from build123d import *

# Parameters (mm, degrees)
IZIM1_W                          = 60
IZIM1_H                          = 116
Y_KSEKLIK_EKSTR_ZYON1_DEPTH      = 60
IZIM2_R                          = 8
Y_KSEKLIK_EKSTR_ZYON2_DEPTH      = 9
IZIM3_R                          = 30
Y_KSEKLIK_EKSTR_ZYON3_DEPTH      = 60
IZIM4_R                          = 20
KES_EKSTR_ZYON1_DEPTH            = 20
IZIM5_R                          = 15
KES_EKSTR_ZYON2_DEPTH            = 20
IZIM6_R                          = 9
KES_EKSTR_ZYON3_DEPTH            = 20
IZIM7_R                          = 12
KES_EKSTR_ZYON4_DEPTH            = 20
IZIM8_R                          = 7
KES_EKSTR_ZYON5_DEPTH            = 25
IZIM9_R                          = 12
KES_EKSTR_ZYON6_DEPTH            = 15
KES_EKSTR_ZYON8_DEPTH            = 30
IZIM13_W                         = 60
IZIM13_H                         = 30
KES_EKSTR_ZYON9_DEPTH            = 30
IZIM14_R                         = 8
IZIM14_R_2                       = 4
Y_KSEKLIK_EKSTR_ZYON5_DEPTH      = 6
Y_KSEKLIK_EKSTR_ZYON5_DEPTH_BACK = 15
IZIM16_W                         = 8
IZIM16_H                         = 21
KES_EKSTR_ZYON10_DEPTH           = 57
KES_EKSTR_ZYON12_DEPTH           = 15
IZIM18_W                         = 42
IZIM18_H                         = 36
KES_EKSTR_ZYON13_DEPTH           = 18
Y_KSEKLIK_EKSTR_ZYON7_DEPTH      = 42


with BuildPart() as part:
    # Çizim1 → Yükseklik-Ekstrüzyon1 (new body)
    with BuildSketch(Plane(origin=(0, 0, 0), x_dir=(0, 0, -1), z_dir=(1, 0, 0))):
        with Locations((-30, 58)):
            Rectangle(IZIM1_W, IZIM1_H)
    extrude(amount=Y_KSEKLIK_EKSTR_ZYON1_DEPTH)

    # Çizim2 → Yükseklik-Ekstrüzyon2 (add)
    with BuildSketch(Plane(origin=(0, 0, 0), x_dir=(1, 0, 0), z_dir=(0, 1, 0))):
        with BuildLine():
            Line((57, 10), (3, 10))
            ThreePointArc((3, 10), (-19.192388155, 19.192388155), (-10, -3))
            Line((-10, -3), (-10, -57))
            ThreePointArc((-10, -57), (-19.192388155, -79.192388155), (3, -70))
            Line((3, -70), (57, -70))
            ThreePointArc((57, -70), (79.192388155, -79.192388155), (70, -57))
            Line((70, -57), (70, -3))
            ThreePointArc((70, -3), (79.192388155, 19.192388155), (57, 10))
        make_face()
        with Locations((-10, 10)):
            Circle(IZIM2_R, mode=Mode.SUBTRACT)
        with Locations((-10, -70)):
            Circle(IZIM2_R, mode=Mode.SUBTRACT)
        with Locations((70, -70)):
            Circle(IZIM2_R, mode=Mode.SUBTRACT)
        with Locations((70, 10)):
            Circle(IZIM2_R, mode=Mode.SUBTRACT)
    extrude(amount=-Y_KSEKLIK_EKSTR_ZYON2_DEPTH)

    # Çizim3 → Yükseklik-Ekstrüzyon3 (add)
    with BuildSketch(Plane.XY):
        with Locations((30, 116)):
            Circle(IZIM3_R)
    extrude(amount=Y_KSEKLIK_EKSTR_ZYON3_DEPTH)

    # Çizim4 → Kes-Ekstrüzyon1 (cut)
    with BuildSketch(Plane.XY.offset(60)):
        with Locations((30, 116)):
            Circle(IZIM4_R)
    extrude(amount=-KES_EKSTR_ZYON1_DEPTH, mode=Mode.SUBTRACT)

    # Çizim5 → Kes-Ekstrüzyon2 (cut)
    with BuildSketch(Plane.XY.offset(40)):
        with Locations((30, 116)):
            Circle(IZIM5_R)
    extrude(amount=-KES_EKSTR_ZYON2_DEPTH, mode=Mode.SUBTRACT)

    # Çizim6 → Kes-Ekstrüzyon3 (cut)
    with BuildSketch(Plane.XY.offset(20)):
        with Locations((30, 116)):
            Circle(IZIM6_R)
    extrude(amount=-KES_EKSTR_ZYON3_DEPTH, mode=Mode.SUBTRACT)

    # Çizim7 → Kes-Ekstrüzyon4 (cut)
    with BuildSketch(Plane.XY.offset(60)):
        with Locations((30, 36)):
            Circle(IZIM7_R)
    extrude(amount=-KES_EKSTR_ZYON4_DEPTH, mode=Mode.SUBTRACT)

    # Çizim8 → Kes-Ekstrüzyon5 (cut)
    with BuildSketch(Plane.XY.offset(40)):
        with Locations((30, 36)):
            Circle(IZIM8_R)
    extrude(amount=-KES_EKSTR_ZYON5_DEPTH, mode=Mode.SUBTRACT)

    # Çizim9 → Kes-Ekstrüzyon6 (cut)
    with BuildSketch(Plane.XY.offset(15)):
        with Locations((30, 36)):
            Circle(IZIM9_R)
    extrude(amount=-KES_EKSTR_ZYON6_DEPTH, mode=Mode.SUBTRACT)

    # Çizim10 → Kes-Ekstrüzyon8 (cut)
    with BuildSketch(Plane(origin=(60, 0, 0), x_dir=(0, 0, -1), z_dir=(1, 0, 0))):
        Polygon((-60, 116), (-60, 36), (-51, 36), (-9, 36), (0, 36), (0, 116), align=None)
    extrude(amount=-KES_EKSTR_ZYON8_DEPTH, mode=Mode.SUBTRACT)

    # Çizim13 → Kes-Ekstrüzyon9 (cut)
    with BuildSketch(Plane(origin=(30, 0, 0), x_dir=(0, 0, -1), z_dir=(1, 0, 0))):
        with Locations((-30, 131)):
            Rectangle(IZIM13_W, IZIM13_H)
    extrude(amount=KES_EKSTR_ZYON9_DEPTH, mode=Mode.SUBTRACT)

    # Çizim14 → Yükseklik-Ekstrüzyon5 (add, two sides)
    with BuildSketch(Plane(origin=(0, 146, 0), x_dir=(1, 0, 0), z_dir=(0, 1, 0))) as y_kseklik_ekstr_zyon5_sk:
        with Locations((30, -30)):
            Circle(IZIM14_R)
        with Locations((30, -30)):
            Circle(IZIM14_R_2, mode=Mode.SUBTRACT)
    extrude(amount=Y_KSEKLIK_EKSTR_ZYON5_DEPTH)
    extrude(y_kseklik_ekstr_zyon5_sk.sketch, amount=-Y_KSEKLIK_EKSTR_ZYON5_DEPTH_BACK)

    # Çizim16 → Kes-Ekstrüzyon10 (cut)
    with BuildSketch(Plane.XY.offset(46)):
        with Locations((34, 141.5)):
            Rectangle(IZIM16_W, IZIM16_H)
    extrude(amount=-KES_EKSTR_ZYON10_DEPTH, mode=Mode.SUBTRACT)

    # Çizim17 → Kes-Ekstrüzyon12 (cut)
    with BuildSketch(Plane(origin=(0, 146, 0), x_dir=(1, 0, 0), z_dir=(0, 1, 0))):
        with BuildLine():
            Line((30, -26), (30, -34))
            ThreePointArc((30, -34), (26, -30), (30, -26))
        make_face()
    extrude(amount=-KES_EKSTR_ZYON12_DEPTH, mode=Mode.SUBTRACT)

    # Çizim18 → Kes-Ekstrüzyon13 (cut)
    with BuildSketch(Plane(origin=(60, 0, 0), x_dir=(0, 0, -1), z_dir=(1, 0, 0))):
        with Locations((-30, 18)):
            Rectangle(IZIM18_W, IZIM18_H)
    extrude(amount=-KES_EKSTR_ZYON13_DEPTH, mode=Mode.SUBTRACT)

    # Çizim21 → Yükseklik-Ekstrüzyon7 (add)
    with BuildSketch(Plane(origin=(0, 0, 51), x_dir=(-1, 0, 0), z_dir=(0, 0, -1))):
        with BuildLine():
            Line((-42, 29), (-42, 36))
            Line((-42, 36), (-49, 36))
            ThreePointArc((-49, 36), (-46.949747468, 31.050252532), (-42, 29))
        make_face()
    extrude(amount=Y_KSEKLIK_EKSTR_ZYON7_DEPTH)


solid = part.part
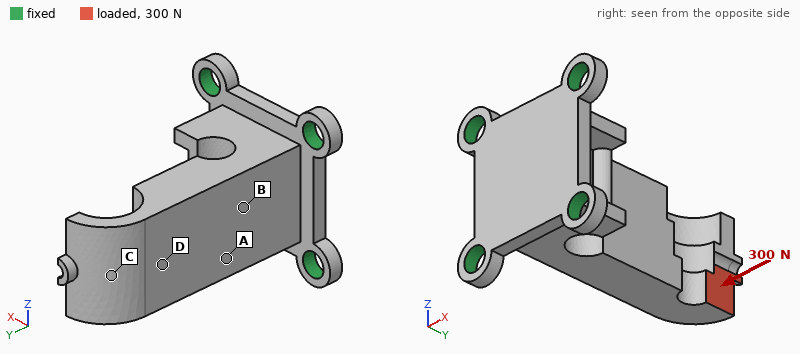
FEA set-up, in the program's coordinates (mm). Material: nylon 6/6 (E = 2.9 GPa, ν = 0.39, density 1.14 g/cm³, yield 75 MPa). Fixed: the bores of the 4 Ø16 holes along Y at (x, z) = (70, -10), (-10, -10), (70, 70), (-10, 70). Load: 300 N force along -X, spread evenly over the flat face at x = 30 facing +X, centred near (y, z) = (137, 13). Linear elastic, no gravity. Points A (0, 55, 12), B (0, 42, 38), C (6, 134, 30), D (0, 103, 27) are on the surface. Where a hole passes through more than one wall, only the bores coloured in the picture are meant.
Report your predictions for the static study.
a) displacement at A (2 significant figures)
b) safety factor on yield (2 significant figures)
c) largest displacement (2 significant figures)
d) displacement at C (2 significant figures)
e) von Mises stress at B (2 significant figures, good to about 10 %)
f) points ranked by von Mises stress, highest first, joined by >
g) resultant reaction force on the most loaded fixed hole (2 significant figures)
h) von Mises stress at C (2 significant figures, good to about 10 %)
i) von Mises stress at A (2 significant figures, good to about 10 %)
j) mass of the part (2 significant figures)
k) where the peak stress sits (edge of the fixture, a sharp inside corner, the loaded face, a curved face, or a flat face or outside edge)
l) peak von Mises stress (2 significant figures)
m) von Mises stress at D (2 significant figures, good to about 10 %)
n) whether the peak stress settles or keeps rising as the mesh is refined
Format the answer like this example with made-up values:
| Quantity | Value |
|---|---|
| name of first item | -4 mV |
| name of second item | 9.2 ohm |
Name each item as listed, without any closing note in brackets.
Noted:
| Quantity | Value |
|---|---|
| displacement at A | 0.33 mm |
| safety factor on yield | 5.3 |
| largest displacement | 1.5 mm |
| displacement at C | 1.2 mm |
| von Mises stress at B | 5.3 MPa |
| points ranked by von Mises stress, highest first, joined by > | B > A > D > C |
| resultant reaction force on the most loaded fixed hole | 380 N |
| von Mises stress at C | 0.96 MPa |
| von Mises stress at A | 3.4 MPa |
| mass of the part | 360 g |
| where the peak stress sits | a curved face |
| peak von Mises stress | 14 MPa |
| von Mises stress at D | 2.3 MPa |
| whether the peak stress settles or keeps rising as the mesh is refined | settles |
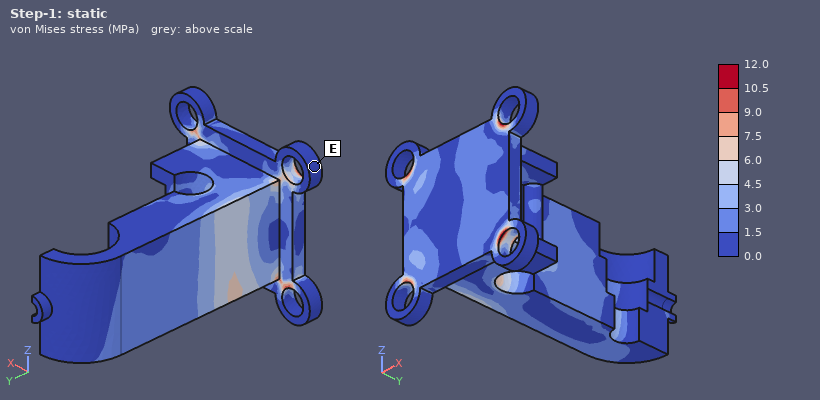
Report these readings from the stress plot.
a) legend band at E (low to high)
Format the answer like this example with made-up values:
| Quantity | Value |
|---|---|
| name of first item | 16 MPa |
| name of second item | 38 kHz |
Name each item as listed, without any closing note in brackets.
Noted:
| Quantity | Value |
|---|---|
| legend band at E | 0.0 to 1.5 MPa |
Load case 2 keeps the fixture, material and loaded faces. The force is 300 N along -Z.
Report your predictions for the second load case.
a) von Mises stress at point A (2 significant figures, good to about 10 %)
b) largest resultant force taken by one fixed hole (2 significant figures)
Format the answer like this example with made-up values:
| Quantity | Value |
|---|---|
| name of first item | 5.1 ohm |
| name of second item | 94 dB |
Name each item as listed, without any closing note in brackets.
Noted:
| Quantity | Value |
|---|---|
| von Mises stress at point A | 1.1 MPa |
| largest resultant force taken by one fixed hole | 470 N |
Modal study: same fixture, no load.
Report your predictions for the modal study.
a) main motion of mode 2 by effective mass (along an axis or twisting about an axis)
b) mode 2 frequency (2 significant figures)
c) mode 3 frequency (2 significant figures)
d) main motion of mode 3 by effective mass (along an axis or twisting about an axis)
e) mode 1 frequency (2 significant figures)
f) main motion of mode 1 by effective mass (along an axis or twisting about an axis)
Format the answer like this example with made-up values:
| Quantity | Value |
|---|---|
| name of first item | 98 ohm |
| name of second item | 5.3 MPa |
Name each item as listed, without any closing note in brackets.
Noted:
| Quantity | Value |
|---|---|
| main motion of mode 2 by effective mass | along Z |
| mode 2 frequency | 440 Hz |
| mode 3 frequency | 1100 Hz |
| main motion of mode 3 by effective mass | along Y |
| mode 1 frequency | 320 Hz |
| main motion of mode 1 by effective mass | along X |
